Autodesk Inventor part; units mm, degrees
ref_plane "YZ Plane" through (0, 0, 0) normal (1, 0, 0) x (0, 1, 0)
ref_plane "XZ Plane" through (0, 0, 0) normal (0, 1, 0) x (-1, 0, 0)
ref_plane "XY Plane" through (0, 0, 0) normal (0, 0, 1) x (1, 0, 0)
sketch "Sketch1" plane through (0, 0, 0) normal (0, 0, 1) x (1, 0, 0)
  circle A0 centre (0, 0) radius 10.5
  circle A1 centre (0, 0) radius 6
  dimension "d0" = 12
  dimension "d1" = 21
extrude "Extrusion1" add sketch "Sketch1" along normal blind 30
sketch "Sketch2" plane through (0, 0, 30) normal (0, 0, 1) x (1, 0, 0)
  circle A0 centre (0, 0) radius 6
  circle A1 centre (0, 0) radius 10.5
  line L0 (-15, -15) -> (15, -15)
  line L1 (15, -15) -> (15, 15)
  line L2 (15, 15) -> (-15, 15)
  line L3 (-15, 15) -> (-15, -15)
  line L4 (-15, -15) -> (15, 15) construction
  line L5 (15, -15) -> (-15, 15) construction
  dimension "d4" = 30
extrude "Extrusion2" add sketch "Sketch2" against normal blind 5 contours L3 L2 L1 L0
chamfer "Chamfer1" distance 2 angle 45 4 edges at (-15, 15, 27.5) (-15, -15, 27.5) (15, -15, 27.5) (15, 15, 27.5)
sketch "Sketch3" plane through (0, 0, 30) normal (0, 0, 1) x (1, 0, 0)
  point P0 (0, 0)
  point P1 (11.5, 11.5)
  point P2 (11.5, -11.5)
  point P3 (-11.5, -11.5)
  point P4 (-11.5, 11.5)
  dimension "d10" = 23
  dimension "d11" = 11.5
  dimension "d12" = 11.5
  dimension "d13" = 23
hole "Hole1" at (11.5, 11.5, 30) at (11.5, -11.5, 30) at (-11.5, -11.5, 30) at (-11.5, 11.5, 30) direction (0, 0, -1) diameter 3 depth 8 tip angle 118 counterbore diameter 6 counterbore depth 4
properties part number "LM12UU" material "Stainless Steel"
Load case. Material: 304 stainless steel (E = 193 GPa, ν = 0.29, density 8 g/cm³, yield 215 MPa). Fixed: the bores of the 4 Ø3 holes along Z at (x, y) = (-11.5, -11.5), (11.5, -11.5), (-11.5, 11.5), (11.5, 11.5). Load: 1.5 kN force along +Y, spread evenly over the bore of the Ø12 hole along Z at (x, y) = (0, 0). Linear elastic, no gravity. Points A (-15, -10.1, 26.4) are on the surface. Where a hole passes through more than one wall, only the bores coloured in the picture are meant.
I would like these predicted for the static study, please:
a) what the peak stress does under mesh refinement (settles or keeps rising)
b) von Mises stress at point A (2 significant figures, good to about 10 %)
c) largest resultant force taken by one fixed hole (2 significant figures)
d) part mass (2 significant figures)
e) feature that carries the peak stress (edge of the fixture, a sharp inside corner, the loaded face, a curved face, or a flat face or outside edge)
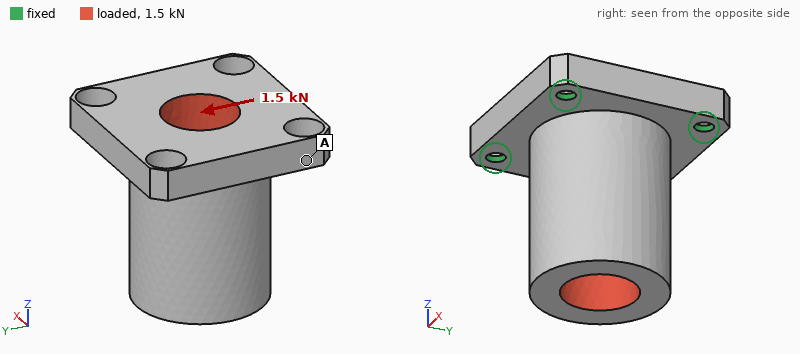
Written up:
keeps rising
22 MPa
520 N
74 g
edge of the fixture
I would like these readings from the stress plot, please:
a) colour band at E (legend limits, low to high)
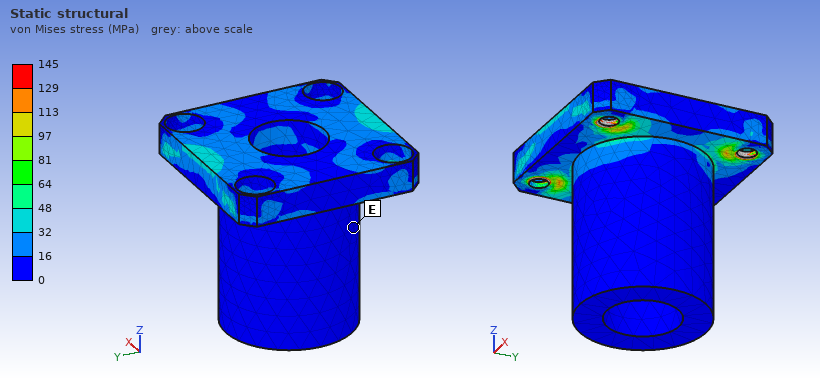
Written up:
0 to 16 MPa
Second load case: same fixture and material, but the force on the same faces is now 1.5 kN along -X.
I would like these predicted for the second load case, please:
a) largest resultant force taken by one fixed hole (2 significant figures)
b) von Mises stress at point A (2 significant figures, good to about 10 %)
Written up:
520 N
36 MPa
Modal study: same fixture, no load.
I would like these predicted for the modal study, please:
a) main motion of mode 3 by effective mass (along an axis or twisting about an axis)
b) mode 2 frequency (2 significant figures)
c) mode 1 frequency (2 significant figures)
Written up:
along Z
7400 Hz
7300 Hz
